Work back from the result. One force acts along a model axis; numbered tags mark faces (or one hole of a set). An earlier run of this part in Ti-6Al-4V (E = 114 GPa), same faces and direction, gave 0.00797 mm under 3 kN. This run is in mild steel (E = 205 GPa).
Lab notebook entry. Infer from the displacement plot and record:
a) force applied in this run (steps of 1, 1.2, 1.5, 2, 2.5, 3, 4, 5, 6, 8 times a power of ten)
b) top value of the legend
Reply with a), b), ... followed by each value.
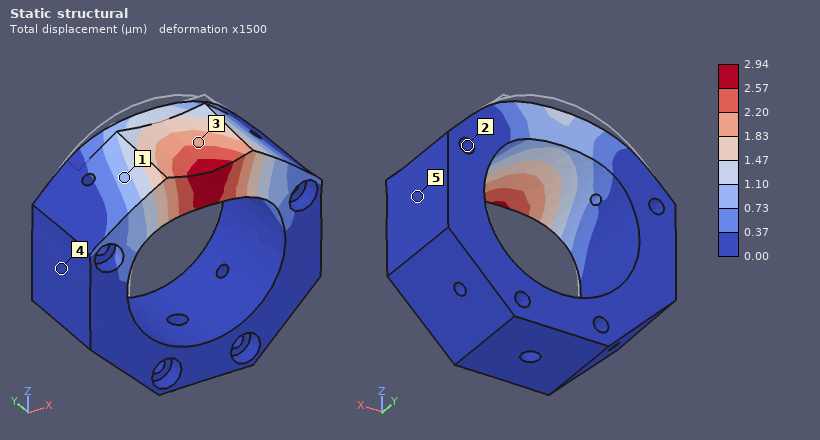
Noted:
a) 2 kN
b) 2.94 µm
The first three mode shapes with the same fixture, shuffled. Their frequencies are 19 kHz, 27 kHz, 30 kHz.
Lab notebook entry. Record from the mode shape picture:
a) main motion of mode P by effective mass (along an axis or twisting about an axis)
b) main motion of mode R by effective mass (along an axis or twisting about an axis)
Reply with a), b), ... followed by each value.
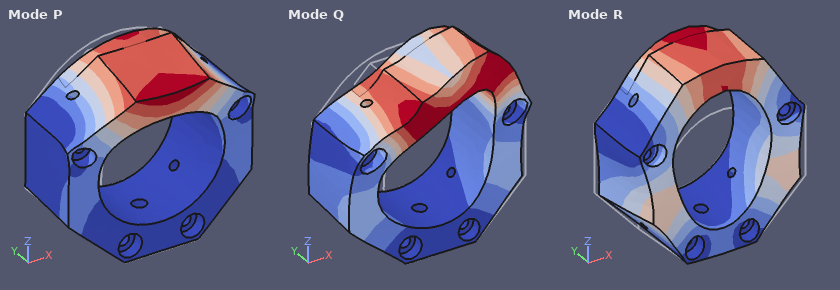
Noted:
a) along Y
b) along Z
